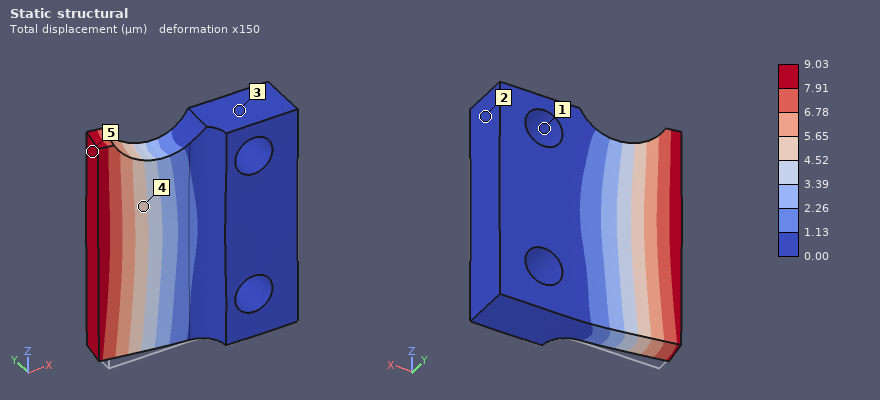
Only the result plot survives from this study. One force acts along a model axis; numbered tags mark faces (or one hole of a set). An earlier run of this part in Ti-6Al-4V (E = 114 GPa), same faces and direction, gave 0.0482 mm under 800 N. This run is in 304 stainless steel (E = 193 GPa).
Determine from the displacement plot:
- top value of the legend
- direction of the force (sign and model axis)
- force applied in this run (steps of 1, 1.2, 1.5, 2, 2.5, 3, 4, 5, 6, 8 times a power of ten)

9.03 µm
+Y
250 N
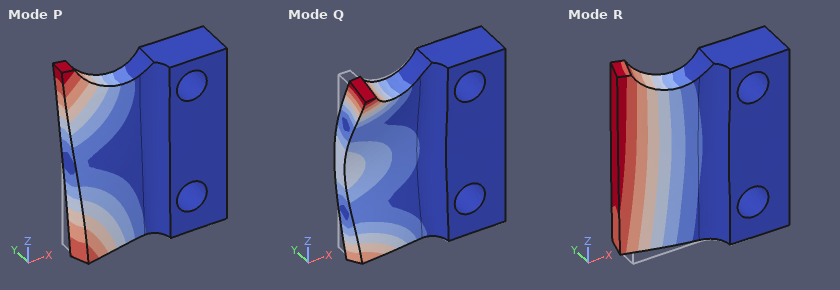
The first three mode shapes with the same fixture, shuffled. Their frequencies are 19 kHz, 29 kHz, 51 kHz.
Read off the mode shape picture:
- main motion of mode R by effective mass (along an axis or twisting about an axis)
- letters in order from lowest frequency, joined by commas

along Y
R, P, Q
